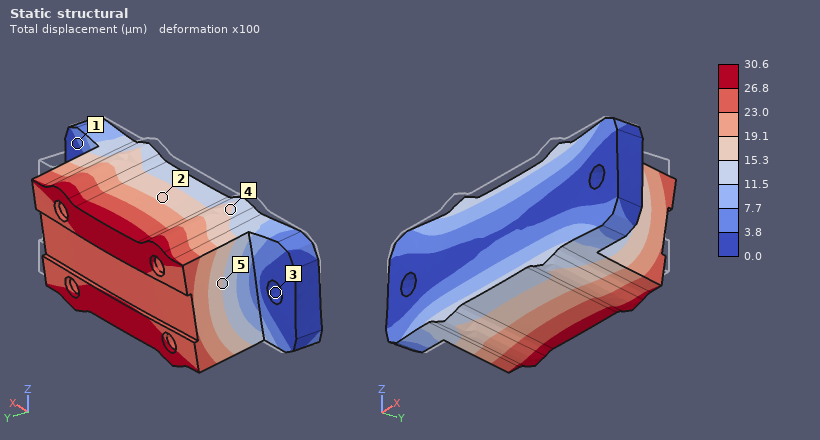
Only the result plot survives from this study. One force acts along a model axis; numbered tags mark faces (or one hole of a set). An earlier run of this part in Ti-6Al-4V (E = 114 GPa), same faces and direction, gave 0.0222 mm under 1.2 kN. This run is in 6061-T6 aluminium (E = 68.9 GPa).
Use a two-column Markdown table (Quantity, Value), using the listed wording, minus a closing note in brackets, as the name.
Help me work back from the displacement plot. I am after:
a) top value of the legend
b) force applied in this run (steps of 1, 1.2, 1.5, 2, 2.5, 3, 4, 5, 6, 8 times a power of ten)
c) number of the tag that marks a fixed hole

| Quantity | Value |
|---|---|
| top value of the legend | 30.6 µm |
| force applied in this run | 1 kN |
| number of the tag that marks a fixed hole | 3 |
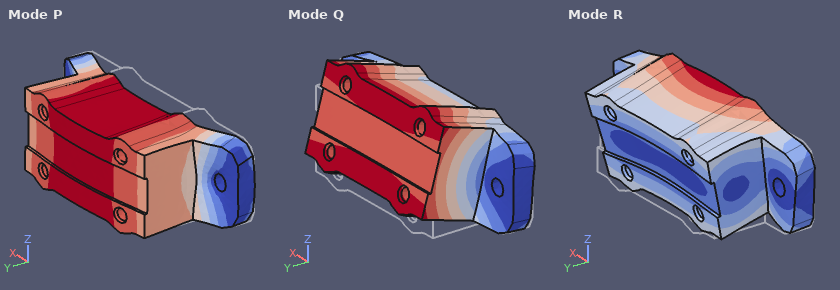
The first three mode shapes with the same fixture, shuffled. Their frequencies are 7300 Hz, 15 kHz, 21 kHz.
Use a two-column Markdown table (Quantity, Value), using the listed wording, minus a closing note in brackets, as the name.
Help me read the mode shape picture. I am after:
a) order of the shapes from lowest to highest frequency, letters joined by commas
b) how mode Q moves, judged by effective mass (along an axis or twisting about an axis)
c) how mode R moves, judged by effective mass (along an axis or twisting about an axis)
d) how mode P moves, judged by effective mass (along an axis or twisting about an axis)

| Quantity | Value |
|---|---|
| order of the shapes from lowest to highest frequency, letters joined by commas | Q, P, R |
| how mode Q moves, judged by effective mass | along Z |
| how mode R moves, judged by effective mass | along Z |
| how mode P moves, judged by effective mass | along Y |
